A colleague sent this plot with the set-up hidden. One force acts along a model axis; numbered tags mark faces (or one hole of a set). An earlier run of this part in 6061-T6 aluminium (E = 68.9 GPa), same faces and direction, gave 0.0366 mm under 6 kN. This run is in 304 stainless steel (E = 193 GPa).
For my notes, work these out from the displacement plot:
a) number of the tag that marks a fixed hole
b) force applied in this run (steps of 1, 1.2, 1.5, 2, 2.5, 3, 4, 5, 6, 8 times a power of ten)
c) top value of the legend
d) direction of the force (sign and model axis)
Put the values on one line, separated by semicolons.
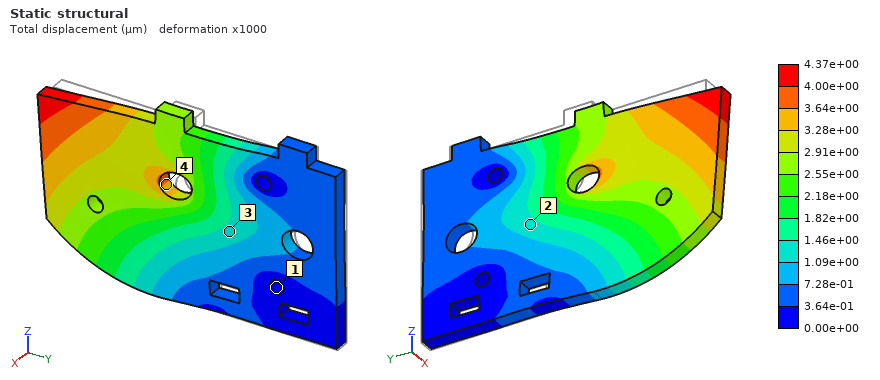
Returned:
1; 2 kN; 4.37e+00 µm; -Y
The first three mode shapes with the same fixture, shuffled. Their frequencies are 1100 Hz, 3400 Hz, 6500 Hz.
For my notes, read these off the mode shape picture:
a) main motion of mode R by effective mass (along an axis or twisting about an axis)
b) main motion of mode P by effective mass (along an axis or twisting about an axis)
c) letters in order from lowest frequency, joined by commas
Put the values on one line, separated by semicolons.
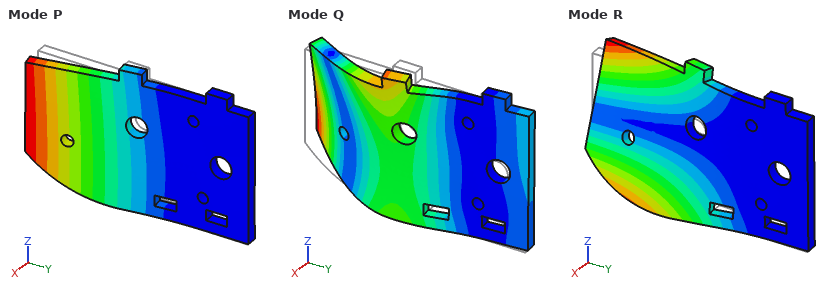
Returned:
twisting about Y; along X; P, R, Q
